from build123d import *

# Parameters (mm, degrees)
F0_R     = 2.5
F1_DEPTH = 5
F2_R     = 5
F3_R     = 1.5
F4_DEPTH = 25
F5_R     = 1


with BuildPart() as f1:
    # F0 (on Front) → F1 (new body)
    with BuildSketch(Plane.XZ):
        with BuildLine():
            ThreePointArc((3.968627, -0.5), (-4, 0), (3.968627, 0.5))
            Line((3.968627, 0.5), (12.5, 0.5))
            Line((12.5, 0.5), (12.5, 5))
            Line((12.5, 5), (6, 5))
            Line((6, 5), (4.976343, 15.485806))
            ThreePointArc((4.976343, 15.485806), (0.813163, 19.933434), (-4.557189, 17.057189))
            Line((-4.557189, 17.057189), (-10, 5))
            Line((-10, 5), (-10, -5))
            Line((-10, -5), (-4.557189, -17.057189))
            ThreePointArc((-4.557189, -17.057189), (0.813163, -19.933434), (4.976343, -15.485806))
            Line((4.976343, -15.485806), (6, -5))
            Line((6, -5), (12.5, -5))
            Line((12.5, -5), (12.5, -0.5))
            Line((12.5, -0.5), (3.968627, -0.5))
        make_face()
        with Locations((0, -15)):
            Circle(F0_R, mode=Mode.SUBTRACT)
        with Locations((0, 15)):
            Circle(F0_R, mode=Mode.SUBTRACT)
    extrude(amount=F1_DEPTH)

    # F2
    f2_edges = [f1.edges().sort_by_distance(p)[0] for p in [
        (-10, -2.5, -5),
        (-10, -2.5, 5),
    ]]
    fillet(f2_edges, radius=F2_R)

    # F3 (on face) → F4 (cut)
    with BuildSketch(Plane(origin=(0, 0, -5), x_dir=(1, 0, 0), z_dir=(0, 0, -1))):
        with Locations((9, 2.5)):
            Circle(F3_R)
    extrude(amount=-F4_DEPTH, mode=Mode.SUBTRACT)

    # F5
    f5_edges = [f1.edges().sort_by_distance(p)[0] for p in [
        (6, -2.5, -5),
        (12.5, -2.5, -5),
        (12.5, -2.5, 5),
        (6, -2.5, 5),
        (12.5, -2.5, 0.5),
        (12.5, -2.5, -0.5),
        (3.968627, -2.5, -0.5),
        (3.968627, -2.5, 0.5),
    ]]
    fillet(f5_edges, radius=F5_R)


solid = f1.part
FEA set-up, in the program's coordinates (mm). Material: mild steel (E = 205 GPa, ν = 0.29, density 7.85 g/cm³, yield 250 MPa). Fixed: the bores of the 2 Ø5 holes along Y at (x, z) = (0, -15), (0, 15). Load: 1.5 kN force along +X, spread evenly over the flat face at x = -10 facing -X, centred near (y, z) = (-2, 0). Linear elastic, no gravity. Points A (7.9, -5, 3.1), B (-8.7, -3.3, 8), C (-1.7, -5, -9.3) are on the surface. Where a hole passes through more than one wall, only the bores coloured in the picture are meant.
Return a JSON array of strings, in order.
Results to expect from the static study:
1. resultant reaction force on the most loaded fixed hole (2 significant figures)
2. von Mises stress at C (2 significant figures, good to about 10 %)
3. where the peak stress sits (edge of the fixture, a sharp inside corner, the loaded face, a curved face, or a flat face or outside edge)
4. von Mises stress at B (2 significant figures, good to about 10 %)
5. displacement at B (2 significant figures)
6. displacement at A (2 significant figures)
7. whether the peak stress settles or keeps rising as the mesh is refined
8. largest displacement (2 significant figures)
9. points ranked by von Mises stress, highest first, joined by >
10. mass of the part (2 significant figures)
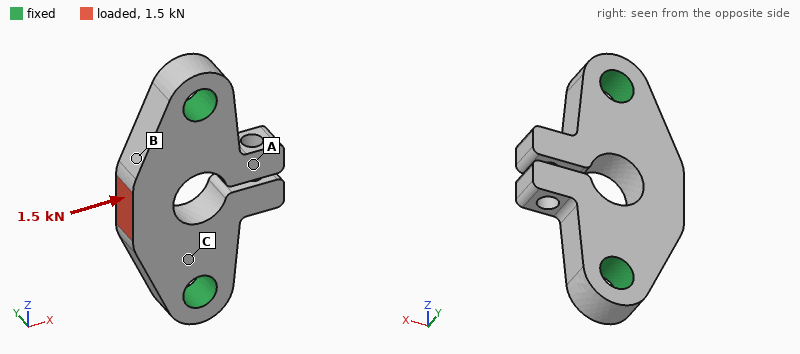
["1.1 kN", "32 MPa", "edge of the fixture", "15 MPa", "1.8 µm", "2.9 µm", "keeps rising", "4.3 µm", "C > B > A", "18 g"]
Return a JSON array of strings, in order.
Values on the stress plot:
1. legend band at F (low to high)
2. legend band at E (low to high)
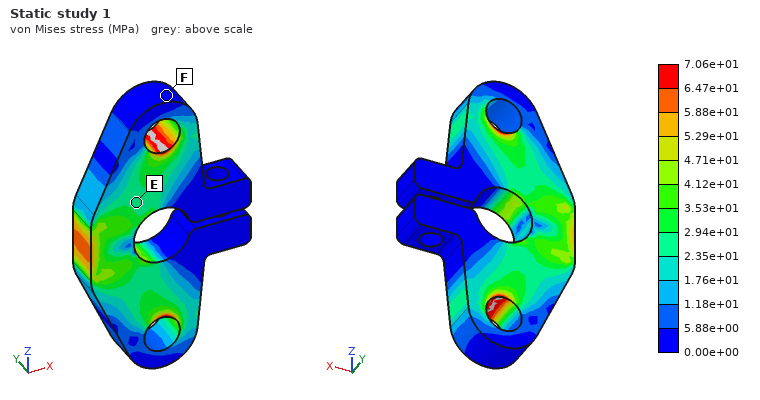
["0.00e+00 to 5.88e+00 MPa", "2.35e+01 to 2.94e+01 MPa"]
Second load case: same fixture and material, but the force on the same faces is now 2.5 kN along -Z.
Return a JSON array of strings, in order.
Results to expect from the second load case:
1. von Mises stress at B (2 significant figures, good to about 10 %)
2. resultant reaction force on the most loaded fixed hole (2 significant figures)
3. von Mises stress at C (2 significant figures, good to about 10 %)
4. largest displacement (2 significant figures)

["58 MPa", "1.5 kN", "32 MPa", "4.4 µm"]
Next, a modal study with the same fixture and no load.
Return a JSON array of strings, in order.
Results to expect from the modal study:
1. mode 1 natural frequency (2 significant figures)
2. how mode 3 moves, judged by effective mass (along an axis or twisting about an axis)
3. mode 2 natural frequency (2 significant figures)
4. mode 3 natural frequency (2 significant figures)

["18 kHz", "along Y", "18 kHz", "24 kHz"]
